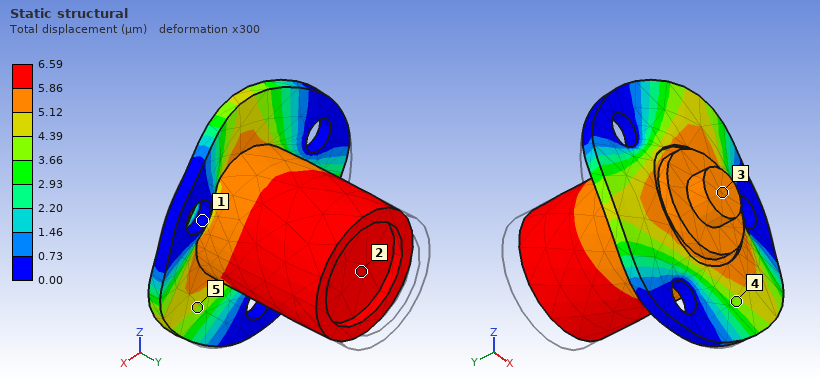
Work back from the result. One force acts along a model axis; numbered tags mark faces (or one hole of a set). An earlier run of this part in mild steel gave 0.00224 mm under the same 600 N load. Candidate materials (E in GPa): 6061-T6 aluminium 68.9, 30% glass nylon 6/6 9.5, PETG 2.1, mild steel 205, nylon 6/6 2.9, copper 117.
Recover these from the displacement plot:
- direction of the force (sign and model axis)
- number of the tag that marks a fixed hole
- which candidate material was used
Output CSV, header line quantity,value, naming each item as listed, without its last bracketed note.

quantity,value
direction of the force,-Y
number of the tag that marks a fixed hole,1
which candidate material was used,6061-T6 aluminium
